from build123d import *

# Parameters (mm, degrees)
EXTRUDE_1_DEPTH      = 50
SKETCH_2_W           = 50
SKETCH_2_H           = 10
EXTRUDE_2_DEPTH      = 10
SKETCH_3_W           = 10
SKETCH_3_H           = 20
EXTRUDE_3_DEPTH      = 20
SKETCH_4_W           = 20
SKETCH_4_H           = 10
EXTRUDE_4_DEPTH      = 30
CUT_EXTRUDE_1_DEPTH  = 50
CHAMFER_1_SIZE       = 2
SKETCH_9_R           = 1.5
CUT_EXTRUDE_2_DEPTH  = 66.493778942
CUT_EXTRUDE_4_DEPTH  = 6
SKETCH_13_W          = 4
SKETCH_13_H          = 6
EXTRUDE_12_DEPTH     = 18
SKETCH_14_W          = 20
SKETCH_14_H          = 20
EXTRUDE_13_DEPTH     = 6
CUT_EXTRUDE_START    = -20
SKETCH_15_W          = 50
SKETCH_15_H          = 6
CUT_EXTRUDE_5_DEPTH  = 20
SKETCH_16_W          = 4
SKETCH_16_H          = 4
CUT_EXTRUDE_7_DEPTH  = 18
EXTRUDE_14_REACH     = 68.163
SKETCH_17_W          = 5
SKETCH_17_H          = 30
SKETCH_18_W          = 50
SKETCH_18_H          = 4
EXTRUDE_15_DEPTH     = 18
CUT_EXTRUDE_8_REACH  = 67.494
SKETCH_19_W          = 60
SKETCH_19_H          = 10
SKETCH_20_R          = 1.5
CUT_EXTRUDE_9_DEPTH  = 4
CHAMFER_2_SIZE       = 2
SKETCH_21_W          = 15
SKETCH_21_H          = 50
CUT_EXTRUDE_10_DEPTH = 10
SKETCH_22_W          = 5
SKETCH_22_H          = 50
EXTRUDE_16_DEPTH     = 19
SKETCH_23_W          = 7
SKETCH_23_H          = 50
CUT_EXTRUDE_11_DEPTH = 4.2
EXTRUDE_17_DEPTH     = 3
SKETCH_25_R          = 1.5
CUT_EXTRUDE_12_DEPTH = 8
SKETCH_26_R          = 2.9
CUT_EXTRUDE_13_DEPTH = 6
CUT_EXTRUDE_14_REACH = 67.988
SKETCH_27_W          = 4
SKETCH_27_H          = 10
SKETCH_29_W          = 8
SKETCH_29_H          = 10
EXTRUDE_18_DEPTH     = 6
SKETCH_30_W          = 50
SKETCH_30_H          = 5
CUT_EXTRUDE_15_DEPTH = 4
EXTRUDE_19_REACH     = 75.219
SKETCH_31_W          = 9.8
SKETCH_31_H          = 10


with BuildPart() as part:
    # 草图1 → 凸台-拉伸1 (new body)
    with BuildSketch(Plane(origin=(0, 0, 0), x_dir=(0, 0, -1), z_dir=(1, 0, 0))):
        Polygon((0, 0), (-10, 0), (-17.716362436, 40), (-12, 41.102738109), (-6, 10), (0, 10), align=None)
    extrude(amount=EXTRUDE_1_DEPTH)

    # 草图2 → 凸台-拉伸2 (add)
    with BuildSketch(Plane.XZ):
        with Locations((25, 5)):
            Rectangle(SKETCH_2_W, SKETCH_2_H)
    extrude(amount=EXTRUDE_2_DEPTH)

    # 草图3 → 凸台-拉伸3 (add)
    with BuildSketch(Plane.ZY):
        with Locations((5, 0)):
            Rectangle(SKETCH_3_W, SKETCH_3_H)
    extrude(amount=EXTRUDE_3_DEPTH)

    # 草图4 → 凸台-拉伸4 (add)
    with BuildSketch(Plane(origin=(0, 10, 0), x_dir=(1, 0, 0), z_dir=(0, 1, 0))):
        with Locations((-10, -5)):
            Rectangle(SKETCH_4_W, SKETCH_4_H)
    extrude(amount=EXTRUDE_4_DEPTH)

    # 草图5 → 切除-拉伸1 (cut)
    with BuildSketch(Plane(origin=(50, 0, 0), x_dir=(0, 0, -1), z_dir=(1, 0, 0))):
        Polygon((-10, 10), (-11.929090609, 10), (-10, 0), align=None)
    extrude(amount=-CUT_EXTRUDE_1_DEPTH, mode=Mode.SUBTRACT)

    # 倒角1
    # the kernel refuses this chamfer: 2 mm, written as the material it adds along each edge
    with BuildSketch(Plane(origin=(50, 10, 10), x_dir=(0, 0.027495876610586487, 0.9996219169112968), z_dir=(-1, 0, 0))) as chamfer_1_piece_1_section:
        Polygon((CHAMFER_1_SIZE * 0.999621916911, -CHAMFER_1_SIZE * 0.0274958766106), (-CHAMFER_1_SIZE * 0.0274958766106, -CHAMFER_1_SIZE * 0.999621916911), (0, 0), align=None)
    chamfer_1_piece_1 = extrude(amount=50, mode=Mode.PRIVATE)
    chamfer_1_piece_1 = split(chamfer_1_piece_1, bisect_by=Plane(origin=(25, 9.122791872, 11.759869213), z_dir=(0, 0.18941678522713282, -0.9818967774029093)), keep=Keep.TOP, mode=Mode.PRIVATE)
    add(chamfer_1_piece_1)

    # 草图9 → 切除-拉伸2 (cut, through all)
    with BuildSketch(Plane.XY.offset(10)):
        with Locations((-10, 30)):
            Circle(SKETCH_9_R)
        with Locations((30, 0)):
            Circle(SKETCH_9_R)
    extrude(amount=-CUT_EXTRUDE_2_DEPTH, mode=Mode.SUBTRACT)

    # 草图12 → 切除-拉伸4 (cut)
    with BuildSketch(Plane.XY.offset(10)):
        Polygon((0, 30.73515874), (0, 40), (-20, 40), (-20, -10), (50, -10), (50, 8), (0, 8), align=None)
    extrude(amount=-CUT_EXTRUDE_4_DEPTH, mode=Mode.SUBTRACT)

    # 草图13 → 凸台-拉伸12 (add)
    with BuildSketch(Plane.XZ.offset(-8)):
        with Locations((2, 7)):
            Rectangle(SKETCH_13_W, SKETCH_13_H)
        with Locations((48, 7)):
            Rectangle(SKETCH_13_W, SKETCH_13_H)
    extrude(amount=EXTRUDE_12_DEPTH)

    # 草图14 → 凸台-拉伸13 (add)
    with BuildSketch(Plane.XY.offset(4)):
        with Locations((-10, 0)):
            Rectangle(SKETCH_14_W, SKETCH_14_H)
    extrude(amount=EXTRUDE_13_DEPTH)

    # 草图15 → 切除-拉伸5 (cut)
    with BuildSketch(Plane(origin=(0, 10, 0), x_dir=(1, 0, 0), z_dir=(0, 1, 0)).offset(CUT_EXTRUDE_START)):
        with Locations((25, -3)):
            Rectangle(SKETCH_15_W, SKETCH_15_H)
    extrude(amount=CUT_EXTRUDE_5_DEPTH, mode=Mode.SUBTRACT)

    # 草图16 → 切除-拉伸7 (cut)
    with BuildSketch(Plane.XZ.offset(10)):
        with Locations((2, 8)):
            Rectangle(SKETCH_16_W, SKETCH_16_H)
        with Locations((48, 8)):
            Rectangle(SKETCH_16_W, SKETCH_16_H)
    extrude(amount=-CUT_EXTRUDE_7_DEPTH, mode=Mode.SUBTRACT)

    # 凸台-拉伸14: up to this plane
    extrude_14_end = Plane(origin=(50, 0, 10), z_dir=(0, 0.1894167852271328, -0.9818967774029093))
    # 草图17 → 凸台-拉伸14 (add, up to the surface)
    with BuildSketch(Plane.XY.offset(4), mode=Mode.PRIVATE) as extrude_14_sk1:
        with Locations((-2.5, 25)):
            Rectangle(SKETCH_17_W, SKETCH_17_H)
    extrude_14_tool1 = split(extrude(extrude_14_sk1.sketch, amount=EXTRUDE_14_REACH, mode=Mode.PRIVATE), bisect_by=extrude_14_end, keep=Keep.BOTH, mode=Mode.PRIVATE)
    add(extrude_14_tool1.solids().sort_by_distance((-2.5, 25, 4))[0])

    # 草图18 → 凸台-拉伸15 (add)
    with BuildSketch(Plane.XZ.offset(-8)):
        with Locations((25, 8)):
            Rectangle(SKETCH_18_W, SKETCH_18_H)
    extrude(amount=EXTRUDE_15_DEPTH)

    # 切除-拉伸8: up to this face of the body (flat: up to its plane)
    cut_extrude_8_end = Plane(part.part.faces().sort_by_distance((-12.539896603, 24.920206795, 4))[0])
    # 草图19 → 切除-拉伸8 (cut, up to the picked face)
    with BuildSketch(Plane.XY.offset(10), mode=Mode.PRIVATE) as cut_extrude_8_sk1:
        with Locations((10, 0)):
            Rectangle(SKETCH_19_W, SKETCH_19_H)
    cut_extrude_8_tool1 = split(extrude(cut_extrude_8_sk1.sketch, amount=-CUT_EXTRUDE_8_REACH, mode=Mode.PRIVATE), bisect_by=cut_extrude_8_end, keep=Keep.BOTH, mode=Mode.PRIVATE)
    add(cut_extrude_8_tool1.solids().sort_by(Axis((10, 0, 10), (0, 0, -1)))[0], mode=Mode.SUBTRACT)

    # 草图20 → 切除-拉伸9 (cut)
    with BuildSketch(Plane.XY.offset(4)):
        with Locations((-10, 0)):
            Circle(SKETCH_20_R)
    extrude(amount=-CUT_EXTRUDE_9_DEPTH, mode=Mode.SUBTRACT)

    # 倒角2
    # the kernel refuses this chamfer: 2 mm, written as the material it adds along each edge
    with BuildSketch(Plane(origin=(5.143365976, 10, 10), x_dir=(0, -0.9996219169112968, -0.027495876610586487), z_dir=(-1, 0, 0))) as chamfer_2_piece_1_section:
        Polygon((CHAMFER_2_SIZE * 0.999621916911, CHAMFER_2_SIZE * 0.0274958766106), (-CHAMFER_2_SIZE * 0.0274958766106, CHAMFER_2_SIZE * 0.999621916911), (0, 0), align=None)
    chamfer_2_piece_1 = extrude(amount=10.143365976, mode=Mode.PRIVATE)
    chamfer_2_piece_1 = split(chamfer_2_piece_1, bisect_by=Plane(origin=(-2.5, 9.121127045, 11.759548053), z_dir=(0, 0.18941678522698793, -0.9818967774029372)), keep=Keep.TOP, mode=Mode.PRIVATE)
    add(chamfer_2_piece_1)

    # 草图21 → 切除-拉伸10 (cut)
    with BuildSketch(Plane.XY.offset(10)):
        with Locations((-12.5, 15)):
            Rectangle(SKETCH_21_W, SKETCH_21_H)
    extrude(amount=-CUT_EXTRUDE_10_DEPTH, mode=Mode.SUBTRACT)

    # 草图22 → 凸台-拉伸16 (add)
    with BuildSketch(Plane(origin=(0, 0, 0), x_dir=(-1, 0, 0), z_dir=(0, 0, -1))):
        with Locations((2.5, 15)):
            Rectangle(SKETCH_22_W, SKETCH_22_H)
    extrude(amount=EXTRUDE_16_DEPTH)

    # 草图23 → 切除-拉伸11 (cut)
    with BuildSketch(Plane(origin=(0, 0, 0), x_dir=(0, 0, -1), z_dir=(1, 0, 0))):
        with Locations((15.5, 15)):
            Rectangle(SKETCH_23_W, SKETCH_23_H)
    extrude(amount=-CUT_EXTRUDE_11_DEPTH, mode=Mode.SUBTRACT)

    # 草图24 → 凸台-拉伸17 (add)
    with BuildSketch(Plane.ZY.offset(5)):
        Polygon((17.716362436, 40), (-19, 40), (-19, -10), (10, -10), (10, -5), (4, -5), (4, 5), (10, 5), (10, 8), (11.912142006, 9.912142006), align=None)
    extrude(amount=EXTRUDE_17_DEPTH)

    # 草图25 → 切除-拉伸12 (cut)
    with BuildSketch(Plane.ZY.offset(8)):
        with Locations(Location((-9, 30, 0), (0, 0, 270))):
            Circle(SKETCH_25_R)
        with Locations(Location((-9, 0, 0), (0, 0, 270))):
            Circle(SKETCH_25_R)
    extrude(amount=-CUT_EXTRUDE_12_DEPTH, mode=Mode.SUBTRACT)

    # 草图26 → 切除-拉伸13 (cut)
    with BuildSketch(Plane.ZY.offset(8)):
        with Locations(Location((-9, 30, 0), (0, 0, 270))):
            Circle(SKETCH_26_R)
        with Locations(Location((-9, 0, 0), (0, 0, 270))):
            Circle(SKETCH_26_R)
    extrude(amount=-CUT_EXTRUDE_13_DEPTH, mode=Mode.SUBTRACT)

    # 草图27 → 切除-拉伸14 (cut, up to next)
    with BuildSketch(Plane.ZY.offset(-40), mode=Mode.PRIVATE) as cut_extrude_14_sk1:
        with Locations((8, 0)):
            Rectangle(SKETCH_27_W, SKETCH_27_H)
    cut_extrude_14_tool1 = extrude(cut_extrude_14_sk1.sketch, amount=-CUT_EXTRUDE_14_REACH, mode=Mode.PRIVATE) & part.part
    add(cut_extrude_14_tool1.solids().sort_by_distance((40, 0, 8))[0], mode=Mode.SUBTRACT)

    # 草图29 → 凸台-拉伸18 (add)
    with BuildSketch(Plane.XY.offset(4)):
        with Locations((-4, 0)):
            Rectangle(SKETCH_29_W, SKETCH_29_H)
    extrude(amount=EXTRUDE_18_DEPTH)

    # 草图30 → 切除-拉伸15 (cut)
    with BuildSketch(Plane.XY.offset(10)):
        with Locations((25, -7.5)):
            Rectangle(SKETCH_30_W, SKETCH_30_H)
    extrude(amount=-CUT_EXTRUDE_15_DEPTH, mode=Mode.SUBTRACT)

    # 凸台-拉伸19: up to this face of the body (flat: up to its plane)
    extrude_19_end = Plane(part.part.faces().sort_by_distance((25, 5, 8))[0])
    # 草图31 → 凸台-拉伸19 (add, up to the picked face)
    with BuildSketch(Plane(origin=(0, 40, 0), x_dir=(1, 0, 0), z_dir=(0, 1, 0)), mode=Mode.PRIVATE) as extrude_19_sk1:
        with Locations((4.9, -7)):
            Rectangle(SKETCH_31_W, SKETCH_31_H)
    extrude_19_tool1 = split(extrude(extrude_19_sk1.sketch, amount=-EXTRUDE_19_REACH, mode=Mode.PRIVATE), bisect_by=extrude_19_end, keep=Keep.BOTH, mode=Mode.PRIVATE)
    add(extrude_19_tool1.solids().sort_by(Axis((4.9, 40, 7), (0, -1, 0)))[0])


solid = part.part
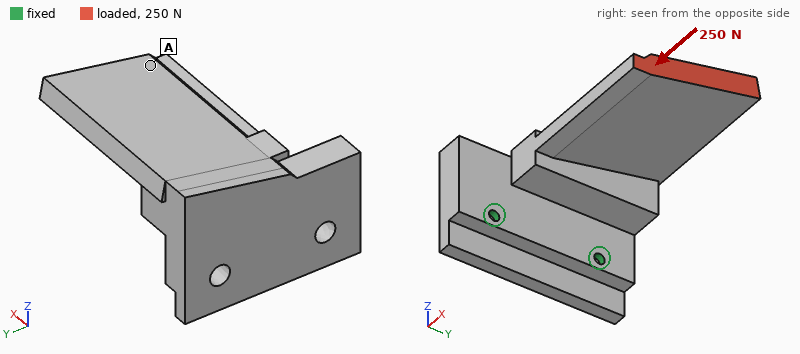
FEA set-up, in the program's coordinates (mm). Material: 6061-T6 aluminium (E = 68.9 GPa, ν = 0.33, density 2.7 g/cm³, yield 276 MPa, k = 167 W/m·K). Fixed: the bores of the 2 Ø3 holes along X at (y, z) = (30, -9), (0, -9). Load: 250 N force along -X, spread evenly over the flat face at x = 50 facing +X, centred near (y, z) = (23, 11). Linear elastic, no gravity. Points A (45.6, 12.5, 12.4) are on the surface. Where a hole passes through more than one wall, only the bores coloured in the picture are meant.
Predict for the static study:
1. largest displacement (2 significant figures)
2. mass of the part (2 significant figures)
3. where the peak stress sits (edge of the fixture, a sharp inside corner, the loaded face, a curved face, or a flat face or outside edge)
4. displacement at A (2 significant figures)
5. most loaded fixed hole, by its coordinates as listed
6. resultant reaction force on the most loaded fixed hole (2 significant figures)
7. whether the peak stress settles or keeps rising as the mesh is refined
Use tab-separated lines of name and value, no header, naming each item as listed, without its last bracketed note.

largest displacement	0.22 mm
mass of the part	63 g
where the peak stress sits	edge of the fixture
displacement at A	0.20 mm
most loaded fixed hole, by its coordinates as listed	(30, -9)
resultant reaction force on the most loaded fixed hole	190 N
whether the peak stress settles or keeps rising as the mesh is refined	keeps rising
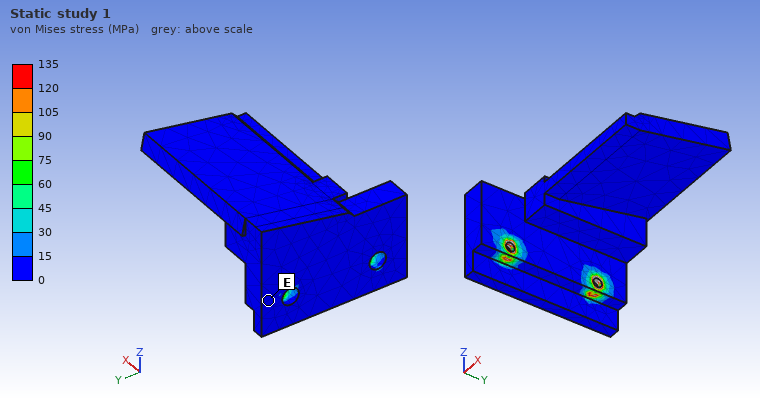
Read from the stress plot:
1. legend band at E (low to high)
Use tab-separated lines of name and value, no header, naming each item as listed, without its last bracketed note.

legend band at E	0 to 15 MPa
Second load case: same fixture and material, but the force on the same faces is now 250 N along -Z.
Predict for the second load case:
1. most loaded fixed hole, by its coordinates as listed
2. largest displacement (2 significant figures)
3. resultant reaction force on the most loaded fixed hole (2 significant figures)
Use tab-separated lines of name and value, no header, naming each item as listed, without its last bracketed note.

most loaded fixed hole, by its coordinates as listed	(30, -9)
largest displacement	0.76 mm
resultant reaction force on the most loaded fixed hole	200 N
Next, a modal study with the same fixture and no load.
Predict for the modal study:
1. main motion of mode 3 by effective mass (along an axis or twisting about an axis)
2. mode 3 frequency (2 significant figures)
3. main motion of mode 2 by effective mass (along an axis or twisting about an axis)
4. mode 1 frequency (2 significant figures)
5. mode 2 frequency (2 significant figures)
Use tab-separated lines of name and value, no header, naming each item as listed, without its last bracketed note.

main motion of mode 3 by effective mass	along X
mode 3 frequency	3800 Hz
main motion of mode 2 by effective mass	along Y
mode 1 frequency	850 Hz
mode 2 frequency	2800 Hz
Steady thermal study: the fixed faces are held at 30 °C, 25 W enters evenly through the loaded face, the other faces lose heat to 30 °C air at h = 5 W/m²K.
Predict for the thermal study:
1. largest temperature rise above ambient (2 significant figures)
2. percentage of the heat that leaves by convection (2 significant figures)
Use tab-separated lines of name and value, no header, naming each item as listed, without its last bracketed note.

largest temperature rise above ambient	49 K
percentage of the heat that leaves by convection	3.5 %
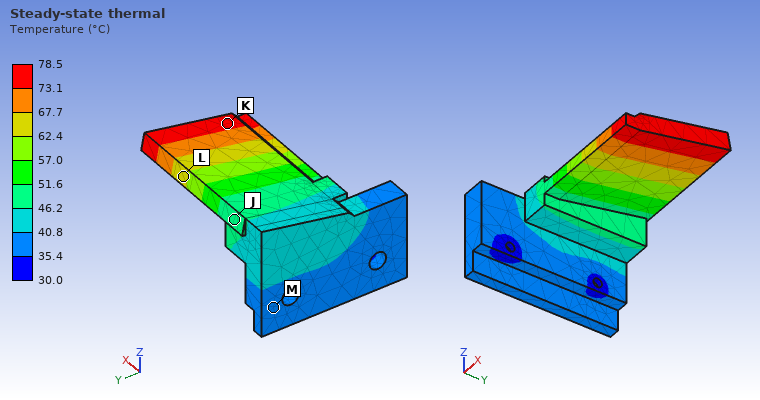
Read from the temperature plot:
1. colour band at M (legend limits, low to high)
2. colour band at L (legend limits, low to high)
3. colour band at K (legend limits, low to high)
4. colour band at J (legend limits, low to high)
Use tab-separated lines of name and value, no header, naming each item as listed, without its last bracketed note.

colour band at M	35.4 to 40.8 °C
colour band at L	62.4 to 67.7 °C
colour band at K	73.1 to 78.5 °C
colour band at J	46.2 to 51.6 °C
